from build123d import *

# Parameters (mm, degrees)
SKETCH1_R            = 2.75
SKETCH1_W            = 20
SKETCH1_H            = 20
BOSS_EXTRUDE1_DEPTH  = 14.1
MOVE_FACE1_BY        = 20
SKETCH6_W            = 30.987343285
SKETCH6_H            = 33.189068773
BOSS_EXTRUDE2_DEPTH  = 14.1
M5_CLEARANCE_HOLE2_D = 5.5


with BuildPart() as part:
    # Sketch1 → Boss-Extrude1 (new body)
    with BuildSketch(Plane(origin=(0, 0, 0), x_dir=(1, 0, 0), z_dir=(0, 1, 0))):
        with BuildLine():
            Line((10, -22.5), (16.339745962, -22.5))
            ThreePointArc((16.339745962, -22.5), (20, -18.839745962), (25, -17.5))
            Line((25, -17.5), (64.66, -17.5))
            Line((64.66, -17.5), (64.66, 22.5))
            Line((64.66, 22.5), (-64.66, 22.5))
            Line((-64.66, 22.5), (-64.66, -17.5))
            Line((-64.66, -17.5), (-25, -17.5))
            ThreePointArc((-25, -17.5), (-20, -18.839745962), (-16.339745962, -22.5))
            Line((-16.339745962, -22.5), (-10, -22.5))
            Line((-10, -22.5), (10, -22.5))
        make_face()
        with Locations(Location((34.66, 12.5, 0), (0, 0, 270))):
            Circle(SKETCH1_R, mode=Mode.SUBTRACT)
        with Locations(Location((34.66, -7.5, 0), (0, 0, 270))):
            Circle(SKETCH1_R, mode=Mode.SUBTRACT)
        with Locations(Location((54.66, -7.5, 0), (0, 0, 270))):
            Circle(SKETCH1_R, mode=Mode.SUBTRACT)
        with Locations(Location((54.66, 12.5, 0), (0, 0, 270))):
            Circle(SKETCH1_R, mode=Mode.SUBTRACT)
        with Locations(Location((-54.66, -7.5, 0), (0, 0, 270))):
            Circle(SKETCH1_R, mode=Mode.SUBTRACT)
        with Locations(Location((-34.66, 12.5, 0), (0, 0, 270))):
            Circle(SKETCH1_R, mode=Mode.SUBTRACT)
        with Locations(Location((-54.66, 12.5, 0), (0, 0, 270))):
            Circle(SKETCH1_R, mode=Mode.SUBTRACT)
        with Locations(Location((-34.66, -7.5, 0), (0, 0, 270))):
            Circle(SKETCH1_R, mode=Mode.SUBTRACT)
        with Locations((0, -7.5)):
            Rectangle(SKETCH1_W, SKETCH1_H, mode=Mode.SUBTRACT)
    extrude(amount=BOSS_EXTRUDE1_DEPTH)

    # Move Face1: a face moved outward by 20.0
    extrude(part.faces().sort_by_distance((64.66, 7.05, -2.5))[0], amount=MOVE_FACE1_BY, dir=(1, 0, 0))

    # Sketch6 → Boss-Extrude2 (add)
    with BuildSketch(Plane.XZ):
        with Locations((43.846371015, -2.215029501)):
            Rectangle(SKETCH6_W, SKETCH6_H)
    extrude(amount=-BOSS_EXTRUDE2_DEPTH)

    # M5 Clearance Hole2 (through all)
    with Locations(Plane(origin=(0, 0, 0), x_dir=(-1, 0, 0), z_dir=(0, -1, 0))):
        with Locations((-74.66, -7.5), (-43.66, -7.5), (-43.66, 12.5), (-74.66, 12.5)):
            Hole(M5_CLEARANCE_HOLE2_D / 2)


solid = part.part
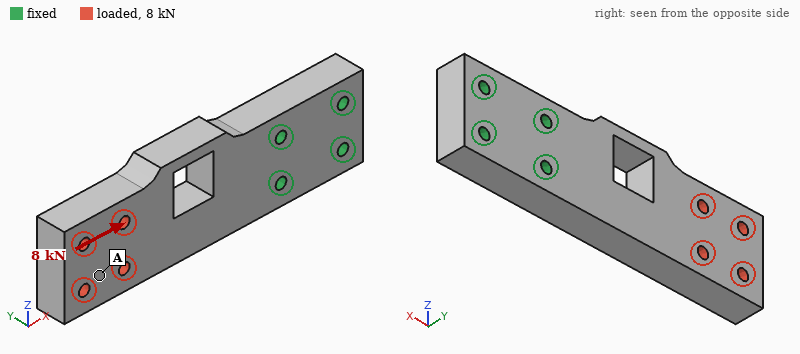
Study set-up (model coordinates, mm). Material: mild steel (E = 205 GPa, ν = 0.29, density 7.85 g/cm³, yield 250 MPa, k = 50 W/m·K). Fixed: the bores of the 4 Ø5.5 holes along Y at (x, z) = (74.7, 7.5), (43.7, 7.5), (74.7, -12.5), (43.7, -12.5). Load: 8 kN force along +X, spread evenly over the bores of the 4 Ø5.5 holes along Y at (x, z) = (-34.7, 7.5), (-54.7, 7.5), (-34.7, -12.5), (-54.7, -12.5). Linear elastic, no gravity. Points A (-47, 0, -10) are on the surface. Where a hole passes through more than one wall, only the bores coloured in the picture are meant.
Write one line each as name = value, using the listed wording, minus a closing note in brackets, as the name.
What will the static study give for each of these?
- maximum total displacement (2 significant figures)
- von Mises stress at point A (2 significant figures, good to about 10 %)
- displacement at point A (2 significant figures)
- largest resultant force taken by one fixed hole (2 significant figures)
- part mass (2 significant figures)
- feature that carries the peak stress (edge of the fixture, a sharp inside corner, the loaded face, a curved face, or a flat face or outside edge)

maximum total displacement = 14 µm
von Mises stress at point A = 7.0 MPa
displacement at point A = 9.8 µm
largest resultant force taken by one fixed hole = 3.7 kN
part mass = 620 g
feature that carries the peak stress = a curved face
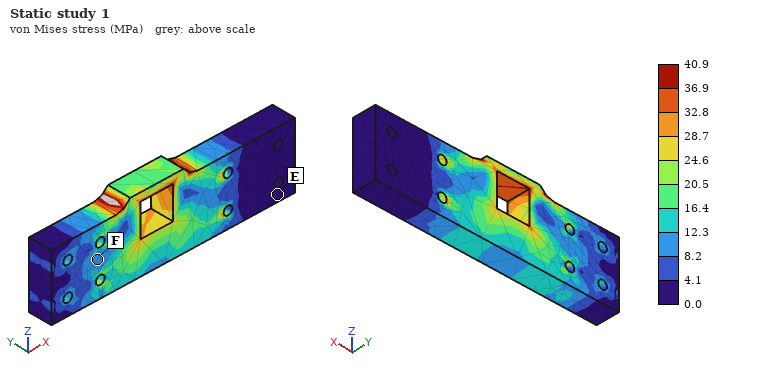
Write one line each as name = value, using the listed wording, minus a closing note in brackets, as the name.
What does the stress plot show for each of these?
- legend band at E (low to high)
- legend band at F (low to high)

legend band at E = 0.0 to 4.1 MPa
legend band at F = 8.2 to 12.3 MPa
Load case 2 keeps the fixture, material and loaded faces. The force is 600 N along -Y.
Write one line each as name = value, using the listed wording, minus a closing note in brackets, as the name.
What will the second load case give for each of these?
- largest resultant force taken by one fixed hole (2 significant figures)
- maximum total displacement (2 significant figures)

largest resultant force taken by one fixed hole = 470 N
maximum total displacement = 0.12 mm
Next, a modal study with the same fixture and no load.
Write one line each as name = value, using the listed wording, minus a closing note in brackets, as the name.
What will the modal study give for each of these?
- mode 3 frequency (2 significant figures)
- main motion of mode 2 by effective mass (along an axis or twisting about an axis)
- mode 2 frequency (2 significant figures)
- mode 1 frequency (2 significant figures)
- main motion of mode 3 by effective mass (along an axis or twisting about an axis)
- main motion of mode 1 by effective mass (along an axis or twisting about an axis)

mode 3 frequency = 4100 Hz
main motion of mode 2 by effective mass = along Z
mode 2 frequency = 2300 Hz
mode 1 frequency = 930 Hz
main motion of mode 3 by effective mass = twisting about X
main motion of mode 1 by effective mass = along Y
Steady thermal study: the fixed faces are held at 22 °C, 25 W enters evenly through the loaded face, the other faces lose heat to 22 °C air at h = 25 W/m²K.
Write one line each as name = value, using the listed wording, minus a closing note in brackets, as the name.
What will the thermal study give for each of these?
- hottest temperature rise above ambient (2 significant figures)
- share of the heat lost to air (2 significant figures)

hottest temperature rise above ambient = 62 K
share of the heat lost to air = 44 %
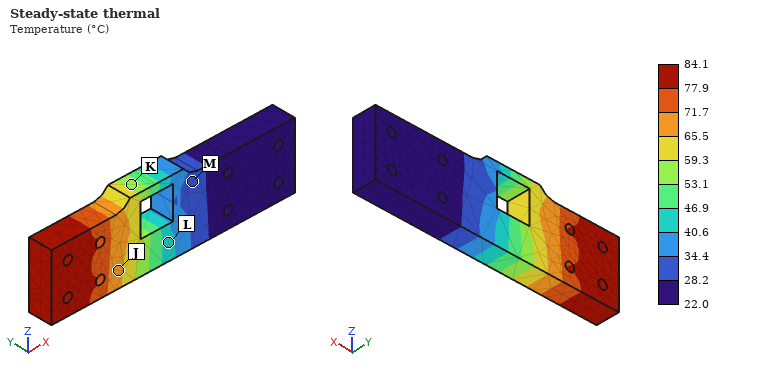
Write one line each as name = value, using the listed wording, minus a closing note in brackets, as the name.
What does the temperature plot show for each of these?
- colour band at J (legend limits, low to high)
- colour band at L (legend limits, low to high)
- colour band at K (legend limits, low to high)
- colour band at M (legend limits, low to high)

colour band at J = 65.5 to 71.7 °C
colour band at L = 40.6 to 46.9 °C
colour band at K = 53.1 to 59.3 °C
colour band at M = 28.2 to 34.4 °C
